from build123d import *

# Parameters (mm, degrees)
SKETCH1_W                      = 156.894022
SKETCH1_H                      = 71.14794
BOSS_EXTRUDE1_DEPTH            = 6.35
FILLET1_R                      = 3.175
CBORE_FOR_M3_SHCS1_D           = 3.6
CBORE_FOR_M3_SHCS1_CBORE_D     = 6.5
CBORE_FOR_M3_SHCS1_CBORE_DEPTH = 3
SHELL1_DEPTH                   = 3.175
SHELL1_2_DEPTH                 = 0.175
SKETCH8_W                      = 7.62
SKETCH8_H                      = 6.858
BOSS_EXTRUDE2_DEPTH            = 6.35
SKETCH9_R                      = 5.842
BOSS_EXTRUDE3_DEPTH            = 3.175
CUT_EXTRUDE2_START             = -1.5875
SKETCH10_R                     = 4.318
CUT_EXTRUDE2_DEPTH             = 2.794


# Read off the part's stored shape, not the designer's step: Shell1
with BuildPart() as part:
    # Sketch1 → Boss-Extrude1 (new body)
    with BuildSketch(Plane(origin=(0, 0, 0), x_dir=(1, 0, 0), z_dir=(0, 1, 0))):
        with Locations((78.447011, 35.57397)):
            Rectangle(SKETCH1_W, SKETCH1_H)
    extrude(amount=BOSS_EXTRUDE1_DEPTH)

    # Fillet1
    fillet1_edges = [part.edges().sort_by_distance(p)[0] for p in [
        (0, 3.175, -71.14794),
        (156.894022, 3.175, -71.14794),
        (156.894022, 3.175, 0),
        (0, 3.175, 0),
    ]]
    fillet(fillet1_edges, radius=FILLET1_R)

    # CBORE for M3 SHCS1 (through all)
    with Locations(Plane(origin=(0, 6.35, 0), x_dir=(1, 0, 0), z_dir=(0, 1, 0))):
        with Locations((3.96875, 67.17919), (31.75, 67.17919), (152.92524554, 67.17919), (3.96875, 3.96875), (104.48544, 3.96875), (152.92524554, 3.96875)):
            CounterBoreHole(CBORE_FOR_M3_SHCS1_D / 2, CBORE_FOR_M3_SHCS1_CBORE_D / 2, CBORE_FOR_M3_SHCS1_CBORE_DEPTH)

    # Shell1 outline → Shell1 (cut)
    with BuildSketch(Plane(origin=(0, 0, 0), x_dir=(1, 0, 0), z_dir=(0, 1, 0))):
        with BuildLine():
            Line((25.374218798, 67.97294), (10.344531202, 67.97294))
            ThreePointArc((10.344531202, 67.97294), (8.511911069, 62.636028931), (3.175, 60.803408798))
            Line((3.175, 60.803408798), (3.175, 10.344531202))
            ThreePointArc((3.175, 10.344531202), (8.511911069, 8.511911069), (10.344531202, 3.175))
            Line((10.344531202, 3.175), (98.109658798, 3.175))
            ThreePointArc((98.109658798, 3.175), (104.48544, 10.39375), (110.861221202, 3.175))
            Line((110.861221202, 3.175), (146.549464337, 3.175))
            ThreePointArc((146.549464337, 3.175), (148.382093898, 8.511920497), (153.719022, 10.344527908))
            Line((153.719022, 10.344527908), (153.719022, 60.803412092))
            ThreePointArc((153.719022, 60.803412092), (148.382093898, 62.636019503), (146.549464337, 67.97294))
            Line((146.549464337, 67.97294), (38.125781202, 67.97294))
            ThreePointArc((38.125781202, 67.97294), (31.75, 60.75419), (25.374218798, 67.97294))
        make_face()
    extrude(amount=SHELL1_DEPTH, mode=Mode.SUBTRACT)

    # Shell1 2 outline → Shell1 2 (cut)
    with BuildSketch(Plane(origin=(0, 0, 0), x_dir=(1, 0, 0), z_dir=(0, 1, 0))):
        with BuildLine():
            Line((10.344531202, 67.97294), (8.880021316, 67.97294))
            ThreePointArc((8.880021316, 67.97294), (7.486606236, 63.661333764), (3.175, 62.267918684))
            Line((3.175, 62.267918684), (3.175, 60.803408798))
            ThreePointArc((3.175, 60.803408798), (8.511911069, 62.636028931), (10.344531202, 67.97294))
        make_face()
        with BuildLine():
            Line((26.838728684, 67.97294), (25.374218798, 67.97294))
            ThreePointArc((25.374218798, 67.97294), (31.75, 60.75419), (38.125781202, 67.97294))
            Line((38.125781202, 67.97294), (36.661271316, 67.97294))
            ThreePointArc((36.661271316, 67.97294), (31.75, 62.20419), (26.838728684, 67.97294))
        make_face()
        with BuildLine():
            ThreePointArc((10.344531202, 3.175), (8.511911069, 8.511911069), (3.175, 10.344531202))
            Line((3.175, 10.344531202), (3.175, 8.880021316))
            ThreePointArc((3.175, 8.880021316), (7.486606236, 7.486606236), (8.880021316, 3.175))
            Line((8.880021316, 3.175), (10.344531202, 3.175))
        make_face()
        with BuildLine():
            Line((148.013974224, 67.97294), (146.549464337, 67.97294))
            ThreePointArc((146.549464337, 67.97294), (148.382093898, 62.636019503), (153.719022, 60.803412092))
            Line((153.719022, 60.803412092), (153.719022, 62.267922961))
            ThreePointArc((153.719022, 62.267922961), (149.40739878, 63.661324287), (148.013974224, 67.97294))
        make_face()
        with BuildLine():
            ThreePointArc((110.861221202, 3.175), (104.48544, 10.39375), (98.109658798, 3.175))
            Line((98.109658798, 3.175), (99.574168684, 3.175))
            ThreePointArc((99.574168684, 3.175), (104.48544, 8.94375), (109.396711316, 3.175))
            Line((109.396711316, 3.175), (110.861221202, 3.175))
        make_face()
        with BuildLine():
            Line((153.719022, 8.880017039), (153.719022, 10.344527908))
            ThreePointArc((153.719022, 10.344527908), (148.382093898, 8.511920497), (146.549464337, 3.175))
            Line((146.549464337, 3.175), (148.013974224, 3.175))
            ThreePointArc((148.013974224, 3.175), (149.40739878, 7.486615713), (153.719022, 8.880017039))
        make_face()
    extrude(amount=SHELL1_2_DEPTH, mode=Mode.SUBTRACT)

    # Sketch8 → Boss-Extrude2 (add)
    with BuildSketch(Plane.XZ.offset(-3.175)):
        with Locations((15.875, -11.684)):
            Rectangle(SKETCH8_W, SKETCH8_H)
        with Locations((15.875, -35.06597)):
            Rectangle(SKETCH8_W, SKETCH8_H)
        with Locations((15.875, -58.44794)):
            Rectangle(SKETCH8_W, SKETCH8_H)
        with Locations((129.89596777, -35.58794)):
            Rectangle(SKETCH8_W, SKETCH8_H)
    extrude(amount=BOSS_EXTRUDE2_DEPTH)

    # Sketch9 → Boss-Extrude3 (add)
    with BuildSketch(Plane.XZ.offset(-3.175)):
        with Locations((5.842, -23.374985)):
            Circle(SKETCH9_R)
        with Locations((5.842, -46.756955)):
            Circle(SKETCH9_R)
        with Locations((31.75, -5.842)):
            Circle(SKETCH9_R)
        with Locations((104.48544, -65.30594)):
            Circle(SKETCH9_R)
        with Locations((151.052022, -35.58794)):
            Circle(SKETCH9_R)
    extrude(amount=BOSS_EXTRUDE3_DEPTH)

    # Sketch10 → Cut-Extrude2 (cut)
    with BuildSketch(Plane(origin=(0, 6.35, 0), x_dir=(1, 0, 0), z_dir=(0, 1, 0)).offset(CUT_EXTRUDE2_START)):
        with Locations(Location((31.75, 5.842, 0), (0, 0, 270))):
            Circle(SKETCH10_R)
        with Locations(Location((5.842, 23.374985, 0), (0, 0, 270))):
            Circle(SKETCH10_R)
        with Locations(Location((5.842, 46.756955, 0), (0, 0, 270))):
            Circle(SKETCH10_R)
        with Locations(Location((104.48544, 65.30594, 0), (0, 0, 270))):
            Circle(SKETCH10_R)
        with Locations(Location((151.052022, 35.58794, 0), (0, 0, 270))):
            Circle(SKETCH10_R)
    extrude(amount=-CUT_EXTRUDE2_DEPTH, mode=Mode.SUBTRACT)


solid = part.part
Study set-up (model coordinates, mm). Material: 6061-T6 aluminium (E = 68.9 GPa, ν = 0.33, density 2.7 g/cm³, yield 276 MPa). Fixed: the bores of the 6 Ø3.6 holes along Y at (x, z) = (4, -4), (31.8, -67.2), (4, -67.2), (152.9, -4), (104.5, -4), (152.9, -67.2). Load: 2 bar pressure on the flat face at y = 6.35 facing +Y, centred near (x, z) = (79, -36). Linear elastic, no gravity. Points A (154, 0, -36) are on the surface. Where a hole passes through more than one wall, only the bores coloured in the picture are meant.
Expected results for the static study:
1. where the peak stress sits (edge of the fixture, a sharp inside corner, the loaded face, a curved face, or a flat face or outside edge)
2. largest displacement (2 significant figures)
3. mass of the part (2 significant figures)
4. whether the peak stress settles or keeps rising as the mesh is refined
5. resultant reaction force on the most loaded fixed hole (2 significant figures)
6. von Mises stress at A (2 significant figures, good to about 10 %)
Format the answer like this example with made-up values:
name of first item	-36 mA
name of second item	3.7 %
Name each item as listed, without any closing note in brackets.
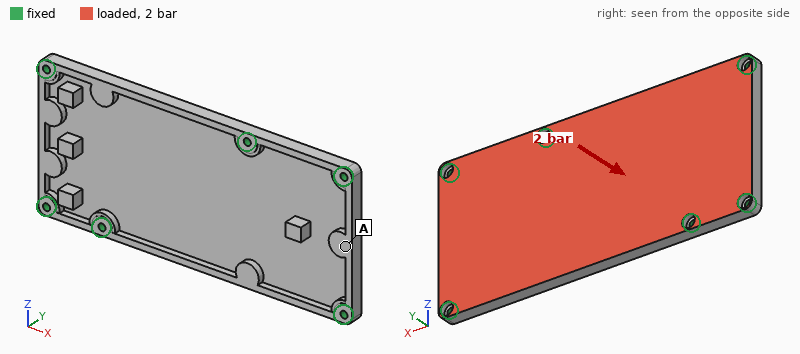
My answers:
where the peak stress sits	edge of the fixture
largest displacement	0.26 mm
mass of the part	110 g
whether the peak stress settles or keeps rising as the mesh is refined	keeps rising
resultant reaction force on the most loaded fixed hole	1.3 kN
von Mises stress at A	13 MPa
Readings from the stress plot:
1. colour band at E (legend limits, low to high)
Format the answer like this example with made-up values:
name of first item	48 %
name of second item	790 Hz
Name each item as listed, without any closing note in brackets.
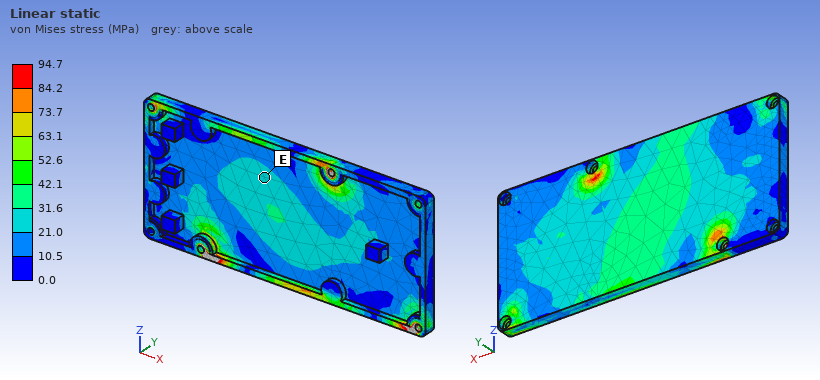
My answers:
colour band at E	21.0 to 31.6 MPa
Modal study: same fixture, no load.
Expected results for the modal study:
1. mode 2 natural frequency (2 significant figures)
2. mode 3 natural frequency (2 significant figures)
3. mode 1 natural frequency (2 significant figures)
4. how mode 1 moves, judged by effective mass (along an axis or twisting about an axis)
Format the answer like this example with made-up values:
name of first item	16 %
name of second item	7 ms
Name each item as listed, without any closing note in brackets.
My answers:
mode 2 natural frequency	2300 Hz
mode 3 natural frequency	3700 Hz
mode 1 natural frequency	1700 Hz
how mode 1 moves, judged by effective mass	along Y
